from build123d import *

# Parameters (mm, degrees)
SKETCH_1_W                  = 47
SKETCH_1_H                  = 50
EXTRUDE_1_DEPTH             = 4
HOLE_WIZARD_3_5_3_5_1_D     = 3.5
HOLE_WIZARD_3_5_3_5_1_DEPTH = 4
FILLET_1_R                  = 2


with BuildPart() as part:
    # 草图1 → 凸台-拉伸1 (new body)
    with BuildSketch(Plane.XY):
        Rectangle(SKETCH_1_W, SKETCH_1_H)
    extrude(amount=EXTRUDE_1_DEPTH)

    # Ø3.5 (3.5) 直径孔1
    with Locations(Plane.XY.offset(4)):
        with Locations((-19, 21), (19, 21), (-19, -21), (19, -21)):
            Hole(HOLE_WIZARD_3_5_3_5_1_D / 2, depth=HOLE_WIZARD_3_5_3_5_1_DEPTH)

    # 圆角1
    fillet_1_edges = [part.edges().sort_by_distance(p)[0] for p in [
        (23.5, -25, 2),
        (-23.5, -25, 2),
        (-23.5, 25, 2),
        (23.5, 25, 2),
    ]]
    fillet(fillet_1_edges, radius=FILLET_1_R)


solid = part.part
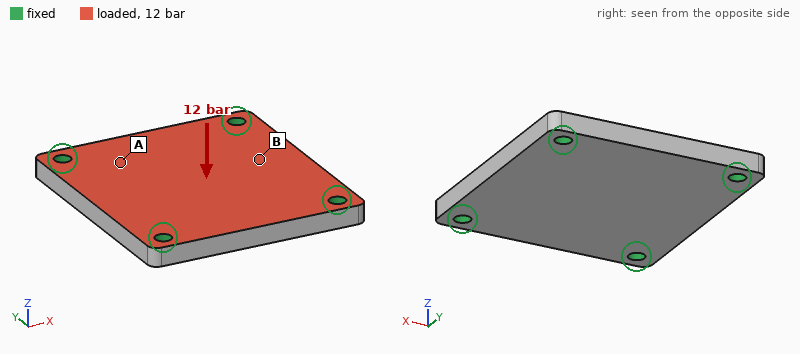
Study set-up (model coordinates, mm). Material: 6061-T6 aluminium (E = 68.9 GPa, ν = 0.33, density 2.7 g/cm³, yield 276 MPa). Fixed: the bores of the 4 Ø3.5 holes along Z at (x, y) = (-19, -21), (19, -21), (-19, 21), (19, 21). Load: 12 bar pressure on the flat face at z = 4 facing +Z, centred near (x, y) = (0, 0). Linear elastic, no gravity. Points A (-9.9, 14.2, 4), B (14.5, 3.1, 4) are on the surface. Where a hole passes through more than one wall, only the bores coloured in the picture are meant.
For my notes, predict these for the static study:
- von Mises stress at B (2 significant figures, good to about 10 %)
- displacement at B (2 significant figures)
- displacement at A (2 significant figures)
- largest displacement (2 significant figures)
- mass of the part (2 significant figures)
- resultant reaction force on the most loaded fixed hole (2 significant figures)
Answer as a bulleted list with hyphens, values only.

- 35 MPa
- 43 µm
- 30 µm
- 58 µm
- 25 g
- 690 N
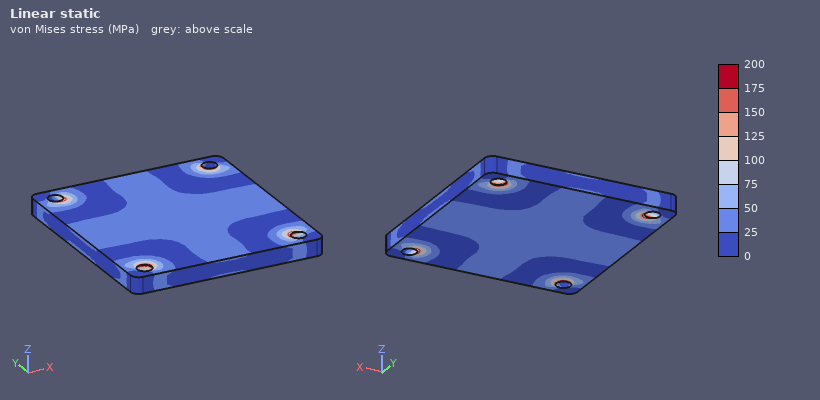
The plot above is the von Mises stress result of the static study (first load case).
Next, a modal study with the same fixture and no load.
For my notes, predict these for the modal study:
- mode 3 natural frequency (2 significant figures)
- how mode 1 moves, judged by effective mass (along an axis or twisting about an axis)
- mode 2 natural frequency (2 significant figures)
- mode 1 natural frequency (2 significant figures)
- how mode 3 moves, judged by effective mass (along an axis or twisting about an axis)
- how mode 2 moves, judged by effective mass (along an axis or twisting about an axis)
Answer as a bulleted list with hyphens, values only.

- 15 kHz
- along Z
- 13 kHz
- 8400 Hz
- twisting about X
- twisting about Y
